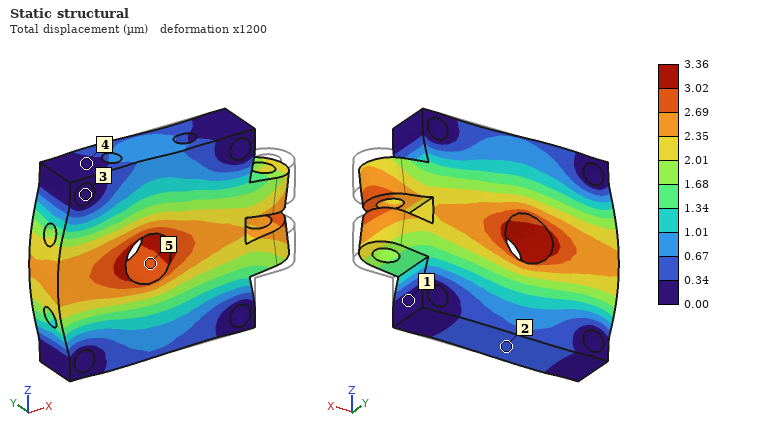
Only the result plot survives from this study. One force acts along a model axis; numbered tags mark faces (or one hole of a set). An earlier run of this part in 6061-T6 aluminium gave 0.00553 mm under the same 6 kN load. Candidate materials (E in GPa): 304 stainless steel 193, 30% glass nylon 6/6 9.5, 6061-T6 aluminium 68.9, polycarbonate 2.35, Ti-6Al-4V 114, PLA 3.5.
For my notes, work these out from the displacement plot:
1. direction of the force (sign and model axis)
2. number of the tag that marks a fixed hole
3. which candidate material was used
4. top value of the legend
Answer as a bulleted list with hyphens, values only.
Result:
- -X
- 3
- Ti-6Al-4V
- 3.36 µm
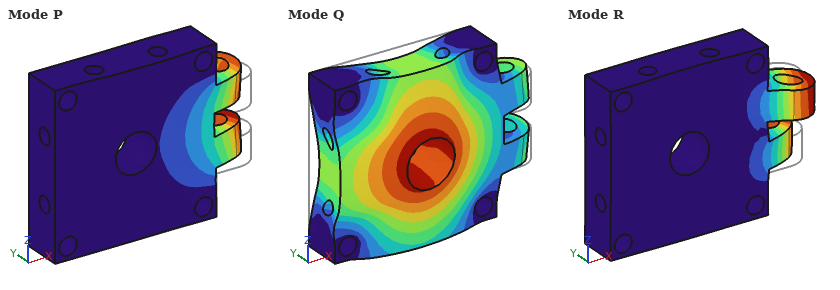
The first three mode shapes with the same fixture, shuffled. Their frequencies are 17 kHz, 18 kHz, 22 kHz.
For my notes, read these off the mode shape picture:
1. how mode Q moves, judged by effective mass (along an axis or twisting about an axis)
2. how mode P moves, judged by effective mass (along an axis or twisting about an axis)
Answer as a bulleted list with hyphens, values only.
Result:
- along Y
- along Y
